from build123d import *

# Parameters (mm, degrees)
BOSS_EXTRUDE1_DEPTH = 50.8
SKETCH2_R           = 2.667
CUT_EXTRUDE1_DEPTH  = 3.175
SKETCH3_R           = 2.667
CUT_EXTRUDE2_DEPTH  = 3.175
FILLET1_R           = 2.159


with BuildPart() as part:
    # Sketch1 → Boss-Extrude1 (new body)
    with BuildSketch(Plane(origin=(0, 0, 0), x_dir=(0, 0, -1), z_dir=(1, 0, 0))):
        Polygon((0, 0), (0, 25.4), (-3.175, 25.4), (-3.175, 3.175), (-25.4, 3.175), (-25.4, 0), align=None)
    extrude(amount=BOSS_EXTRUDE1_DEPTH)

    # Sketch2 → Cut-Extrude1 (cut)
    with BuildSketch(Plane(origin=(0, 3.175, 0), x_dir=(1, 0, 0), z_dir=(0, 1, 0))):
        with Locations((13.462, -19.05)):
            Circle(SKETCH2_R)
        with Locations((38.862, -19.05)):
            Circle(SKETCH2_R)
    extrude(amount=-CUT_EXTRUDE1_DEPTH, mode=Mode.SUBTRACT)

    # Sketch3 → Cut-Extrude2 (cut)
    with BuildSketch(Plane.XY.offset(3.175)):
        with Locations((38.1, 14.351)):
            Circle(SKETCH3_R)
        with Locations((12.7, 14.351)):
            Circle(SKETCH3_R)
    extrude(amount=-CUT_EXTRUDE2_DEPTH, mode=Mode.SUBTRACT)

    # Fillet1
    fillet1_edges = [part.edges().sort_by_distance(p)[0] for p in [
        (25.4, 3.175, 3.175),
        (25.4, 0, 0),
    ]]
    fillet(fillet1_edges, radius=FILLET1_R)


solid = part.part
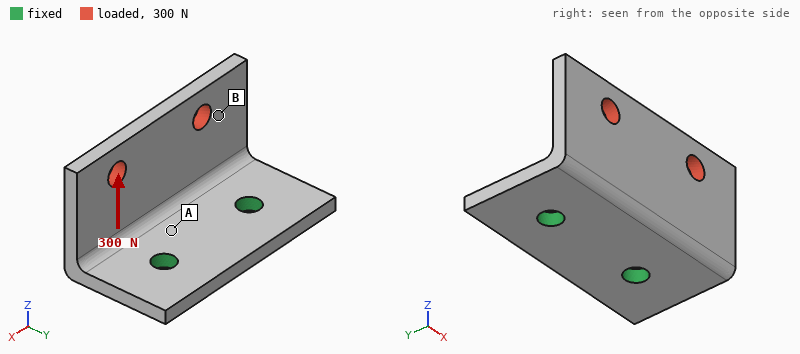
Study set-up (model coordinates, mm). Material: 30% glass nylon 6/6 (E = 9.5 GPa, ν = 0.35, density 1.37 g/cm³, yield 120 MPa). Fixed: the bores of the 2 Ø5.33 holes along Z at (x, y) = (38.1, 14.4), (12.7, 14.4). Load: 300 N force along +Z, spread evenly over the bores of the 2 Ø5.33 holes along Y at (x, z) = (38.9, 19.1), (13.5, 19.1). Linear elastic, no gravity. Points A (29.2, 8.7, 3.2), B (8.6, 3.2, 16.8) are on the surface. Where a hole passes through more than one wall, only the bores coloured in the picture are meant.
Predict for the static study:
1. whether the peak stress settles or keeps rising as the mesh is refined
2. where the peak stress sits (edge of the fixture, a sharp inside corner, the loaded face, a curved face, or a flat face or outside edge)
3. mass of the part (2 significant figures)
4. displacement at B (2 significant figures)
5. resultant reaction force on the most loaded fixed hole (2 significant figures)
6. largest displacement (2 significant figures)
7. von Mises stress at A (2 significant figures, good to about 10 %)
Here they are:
keeps rising
edge of the fixture
10 g
0.27 mm
160 N
0.43 mm
18 MPa
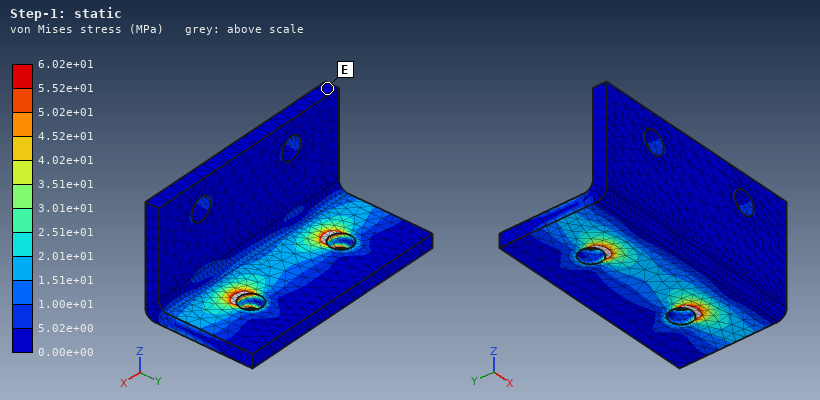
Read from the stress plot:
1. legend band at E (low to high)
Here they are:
0.00e+00 to 5.02e+00 MPa
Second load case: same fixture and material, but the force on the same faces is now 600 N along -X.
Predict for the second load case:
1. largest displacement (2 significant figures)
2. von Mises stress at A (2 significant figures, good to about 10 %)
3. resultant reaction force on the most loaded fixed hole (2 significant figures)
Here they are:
0.63 mm
31 MPa
520 N
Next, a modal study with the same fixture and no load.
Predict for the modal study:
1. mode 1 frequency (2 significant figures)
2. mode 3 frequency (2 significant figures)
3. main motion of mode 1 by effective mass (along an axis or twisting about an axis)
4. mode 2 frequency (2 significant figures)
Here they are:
1500 Hz
4000 Hz
along Y
2300 Hz
